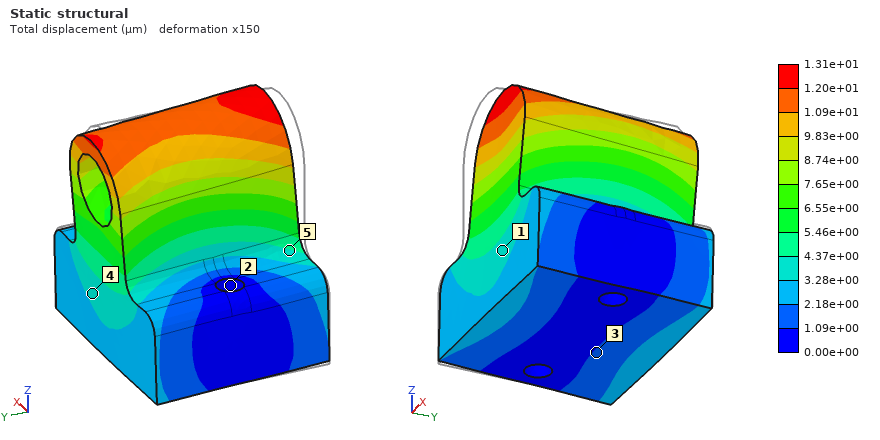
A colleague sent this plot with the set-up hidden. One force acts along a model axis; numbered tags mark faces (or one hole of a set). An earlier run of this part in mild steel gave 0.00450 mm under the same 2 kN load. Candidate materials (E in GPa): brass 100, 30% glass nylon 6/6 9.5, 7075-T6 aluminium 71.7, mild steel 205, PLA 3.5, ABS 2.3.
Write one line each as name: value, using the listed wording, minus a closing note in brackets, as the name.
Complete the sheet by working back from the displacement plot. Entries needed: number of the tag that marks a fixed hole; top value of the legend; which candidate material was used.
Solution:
number of the tag that marks a fixed hole: 2
top value of the legend: 1.31e+01 µm
which candidate material was used: 7075-T6 aluminium
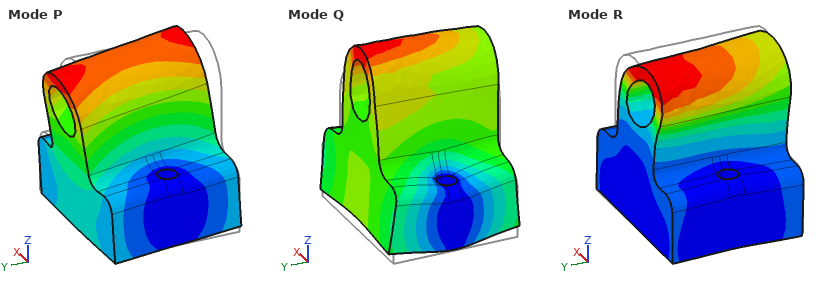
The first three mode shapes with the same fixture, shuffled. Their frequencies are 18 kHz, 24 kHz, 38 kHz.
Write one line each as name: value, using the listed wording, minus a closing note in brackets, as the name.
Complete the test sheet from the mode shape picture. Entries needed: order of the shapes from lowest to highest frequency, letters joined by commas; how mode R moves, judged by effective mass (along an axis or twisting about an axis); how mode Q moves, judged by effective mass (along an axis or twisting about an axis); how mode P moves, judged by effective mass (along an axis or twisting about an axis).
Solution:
order of the shapes from lowest to highest frequency, letters joined by commas: P, R, Q
how mode R moves, judged by effective mass: along X
how mode Q moves, judged by effective mass: along Z
how mode P moves, judged by effective mass: along Y
